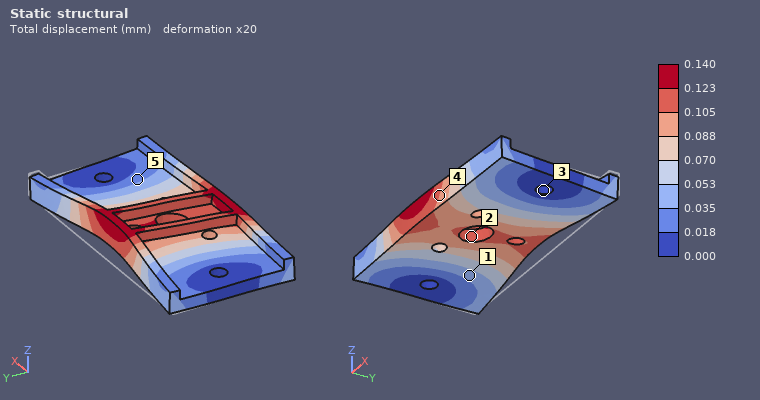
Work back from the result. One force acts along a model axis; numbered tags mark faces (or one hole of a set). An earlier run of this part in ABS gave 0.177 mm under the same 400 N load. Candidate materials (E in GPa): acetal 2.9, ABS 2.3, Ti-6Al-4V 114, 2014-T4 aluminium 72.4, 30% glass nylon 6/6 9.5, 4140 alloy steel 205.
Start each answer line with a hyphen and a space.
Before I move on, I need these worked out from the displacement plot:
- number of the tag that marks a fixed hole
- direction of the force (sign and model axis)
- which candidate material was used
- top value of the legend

- 3
- -Y
- acetal
- 0.140 mm
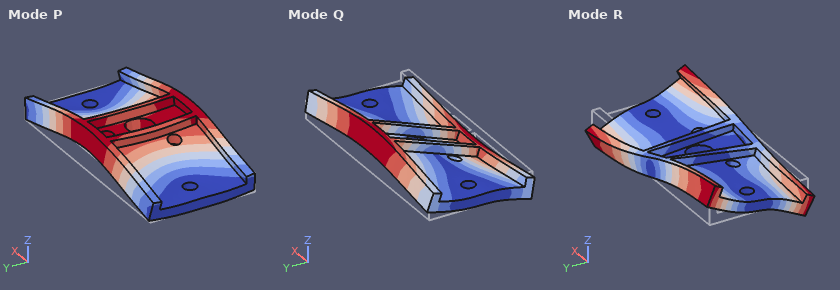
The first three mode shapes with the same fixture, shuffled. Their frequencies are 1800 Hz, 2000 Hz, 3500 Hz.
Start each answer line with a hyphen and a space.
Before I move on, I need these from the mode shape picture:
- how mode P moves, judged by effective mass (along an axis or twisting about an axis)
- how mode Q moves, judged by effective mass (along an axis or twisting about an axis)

- along Z
- twisting about X
